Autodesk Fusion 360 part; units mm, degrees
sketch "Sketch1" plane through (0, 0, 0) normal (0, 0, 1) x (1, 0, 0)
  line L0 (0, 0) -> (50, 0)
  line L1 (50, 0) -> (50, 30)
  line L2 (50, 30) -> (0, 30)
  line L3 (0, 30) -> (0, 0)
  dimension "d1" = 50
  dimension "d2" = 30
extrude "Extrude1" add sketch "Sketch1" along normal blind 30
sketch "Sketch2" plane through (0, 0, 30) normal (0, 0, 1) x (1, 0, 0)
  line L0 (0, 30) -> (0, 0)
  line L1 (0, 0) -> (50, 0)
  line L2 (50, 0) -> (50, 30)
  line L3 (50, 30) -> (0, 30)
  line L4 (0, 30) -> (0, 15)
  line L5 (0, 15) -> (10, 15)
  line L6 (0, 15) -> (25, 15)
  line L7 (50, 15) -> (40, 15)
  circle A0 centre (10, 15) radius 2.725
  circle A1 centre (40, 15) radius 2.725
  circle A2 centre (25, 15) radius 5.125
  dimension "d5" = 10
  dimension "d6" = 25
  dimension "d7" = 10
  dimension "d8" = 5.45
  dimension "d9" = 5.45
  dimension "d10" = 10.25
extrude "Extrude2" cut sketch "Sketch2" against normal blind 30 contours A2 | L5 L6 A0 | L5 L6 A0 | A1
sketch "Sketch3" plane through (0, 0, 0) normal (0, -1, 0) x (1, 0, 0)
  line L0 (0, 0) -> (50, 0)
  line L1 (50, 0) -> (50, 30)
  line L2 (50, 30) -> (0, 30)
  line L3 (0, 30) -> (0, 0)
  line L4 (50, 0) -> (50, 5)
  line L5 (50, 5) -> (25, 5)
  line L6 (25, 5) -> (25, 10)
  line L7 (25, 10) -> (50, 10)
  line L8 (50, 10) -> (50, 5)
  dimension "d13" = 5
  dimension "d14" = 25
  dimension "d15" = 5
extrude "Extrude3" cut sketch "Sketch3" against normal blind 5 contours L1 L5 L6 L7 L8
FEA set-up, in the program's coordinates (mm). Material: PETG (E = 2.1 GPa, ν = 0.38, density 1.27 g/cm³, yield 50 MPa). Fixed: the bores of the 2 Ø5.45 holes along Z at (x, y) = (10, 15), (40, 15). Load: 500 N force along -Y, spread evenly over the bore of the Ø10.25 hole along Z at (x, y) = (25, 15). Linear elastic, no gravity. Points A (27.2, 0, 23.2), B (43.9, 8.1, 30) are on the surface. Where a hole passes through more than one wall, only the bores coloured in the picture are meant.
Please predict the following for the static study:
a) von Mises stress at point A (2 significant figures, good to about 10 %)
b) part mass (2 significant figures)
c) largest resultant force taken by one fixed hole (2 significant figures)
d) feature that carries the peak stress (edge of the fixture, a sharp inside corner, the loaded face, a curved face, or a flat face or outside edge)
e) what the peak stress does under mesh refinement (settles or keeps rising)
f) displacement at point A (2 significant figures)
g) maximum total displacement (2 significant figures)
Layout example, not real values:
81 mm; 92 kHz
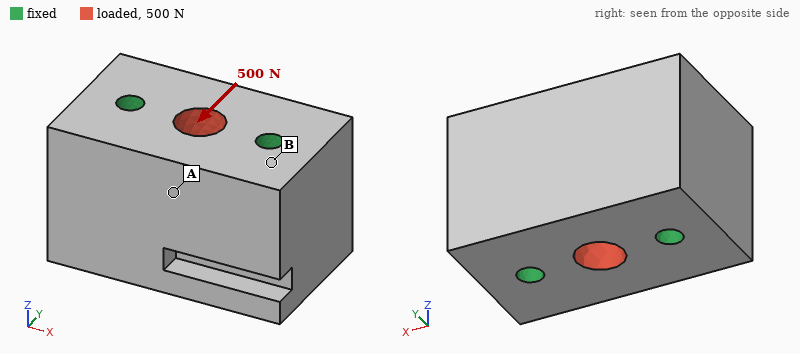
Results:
0.70 MPa; 51 g; 250 N; edge of the fixture; keeps rising; 5.1 µm; 7.6 µm
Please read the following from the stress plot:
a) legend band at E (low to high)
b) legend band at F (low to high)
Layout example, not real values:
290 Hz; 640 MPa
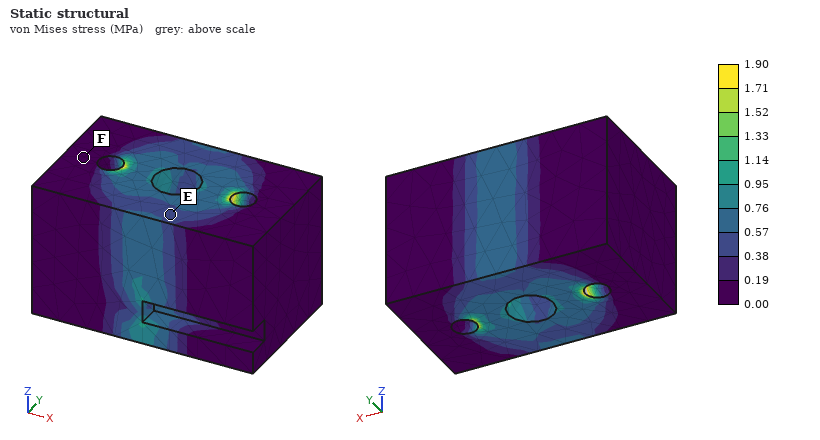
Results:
0.38 to 0.57 MPa; 0.00 to 0.19 MPa
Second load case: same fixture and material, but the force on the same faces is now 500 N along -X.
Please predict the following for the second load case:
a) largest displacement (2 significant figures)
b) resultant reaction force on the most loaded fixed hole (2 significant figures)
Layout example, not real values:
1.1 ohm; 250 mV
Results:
3.6 µm; 250 N
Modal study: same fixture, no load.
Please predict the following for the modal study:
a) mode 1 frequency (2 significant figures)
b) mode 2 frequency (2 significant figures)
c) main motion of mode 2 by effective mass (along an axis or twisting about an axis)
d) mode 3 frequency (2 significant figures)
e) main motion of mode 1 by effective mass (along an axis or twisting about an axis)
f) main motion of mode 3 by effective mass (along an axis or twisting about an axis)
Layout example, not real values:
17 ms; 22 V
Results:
8500 Hz; 8900 Hz; twisting about X; 9400 Hz; twisting about Z; along Z
